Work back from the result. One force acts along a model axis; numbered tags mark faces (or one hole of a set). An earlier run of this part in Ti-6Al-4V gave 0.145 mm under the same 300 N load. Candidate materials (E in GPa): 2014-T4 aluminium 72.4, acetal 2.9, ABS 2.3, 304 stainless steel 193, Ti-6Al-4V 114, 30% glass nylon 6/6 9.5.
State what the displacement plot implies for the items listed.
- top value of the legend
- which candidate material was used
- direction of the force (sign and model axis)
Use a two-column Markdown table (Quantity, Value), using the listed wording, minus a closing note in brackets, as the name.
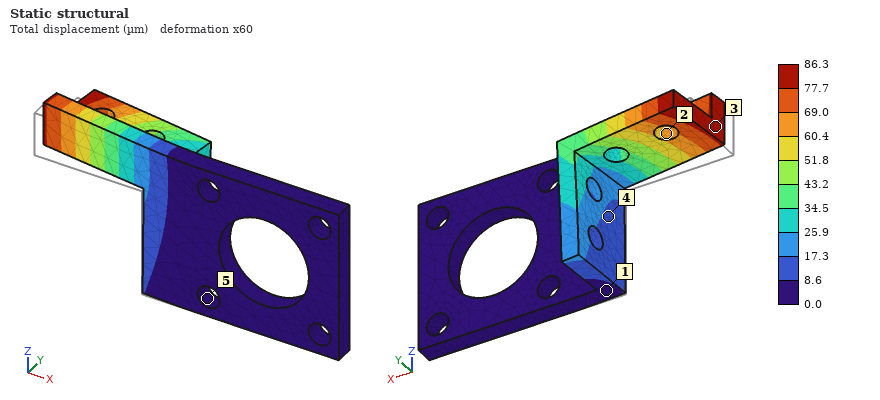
| Quantity | Value |
|---|---|
| top value of the legend | 86.3 µm |
| which candidate material was used | 304 stainless steel |
| direction of the force | +Y |
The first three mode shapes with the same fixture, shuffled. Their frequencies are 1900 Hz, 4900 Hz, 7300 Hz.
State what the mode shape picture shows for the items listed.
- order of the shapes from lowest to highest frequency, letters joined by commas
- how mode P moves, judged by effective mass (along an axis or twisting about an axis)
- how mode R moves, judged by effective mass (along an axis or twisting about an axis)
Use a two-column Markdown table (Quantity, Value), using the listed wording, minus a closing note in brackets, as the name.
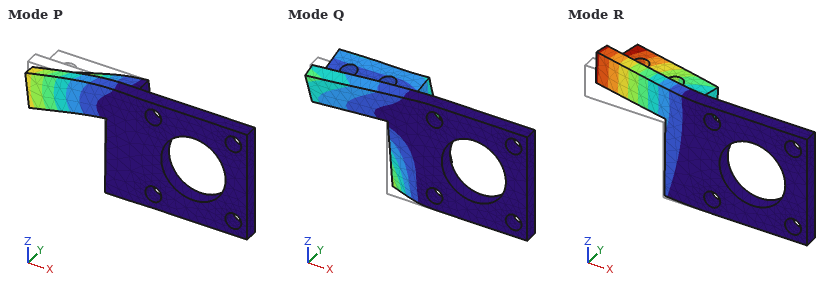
| Quantity | Value |
|---|---|
| order of the shapes from lowest to highest frequency, letters joined by commas | R, P, Q |
| how mode P moves, judged by effective mass | along Z |
| how mode R moves, judged by effective mass | along Y |
